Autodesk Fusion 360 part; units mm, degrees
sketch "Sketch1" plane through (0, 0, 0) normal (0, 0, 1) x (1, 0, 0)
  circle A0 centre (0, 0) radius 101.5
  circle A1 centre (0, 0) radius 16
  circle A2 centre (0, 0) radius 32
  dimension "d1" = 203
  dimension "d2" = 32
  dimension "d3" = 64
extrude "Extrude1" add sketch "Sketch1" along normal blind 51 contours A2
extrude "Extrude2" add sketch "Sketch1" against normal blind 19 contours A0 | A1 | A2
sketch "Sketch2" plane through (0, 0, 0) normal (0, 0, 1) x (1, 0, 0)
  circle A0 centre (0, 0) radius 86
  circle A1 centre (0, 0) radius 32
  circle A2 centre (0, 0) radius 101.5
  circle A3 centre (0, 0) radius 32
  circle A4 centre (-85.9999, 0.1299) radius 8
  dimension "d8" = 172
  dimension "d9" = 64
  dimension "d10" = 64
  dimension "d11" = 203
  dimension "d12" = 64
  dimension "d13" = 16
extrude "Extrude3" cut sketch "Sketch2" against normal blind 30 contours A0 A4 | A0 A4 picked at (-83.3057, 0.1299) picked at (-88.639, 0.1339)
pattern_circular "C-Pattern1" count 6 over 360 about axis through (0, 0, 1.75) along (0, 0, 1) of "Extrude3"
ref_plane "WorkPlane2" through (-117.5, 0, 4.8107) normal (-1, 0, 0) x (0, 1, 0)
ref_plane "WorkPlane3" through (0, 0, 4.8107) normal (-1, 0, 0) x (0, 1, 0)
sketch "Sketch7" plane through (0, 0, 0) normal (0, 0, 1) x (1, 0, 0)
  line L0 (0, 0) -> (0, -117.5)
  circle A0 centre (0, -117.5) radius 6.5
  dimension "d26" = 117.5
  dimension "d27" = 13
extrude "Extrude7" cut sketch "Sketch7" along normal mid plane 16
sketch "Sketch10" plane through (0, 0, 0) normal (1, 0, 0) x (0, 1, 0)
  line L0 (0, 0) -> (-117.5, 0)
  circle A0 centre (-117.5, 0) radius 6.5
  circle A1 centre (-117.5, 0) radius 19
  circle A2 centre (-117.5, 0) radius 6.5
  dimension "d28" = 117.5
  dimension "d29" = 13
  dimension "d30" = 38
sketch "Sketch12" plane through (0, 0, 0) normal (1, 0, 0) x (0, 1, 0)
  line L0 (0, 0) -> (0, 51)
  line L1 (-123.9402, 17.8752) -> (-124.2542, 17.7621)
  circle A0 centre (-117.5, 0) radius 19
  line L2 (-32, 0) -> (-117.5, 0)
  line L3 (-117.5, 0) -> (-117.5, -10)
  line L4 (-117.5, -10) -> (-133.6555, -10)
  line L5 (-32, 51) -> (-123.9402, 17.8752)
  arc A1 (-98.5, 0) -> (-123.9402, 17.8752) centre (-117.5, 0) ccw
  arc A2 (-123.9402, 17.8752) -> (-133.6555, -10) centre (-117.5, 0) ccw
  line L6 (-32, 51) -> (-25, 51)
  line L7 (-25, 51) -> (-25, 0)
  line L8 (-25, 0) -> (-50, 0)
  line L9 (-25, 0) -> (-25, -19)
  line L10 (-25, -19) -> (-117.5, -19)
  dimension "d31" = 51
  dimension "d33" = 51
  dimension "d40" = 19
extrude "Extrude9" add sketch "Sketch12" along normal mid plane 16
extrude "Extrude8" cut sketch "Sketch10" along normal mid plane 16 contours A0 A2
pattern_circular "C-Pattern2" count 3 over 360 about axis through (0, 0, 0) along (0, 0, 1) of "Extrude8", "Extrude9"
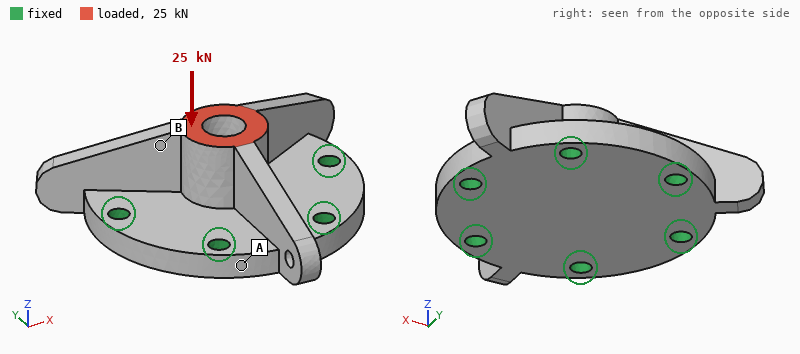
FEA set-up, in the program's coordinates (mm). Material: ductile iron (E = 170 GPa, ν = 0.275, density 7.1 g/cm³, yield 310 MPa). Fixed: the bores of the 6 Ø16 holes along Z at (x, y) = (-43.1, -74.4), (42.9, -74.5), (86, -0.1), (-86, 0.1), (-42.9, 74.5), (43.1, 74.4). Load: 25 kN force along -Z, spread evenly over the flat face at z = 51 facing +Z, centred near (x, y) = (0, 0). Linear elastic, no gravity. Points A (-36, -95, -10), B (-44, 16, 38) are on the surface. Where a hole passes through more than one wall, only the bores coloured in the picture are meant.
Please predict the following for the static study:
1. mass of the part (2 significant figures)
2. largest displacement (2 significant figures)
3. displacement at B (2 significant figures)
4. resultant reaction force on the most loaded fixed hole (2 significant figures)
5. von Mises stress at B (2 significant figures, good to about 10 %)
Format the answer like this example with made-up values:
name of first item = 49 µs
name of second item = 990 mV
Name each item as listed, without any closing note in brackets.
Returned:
mass of the part = 6.4 kg
largest displacement = 13 µm
displacement at B = 8.7 µm
resultant reaction force on the most loaded fixed hole = 4.4 kN
von Mises stress at B = 9.4 MPa
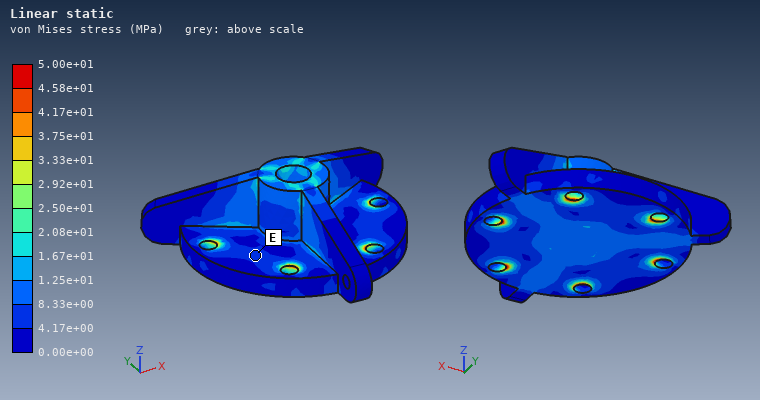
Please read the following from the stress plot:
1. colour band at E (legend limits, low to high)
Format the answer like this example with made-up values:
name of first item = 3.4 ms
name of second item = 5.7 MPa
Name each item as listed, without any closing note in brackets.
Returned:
colour band at E = 4.17e+00 to 8.33e+00 MPa
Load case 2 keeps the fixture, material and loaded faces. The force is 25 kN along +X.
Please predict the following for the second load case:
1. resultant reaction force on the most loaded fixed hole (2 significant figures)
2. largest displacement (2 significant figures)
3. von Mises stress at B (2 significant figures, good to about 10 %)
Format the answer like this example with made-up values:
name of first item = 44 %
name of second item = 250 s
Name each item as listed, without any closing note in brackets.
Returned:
resultant reaction force on the most loaded fixed hole = 8.9 kN
largest displacement = 31 µm
von Mises stress at B = 23 MPa
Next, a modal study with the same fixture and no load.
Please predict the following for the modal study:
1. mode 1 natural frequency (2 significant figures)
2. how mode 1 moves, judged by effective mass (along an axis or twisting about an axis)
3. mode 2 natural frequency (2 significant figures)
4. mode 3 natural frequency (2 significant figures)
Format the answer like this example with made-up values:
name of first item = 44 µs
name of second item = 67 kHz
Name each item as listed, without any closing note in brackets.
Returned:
mode 1 natural frequency = 4800 Hz
how mode 1 moves, judged by effective mass = along Z
mode 2 natural frequency = 5200 Hz
mode 3 natural frequency = 5200 Hz
